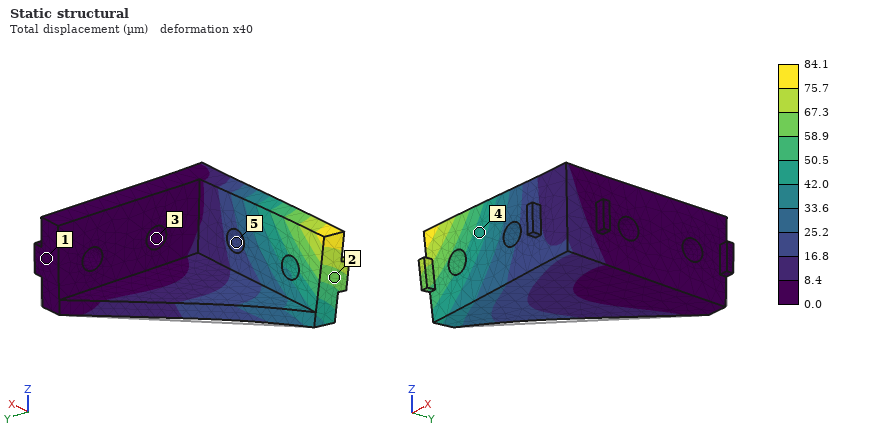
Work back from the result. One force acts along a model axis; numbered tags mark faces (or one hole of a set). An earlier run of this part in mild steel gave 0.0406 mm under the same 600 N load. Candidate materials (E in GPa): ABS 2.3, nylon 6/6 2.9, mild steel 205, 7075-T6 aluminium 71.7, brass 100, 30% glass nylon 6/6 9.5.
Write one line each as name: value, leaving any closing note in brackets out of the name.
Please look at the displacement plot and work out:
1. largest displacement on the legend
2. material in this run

largest displacement on the legend: 84.1 µm
material in this run: brass
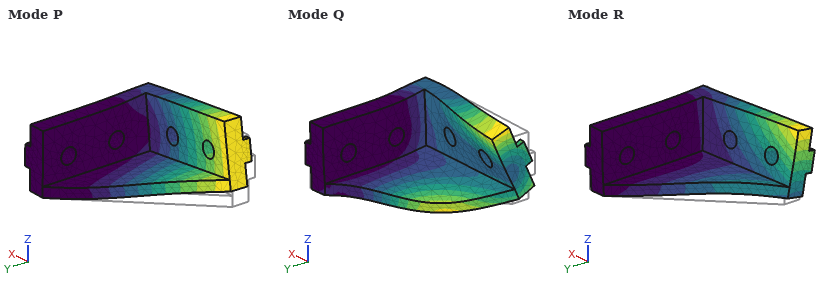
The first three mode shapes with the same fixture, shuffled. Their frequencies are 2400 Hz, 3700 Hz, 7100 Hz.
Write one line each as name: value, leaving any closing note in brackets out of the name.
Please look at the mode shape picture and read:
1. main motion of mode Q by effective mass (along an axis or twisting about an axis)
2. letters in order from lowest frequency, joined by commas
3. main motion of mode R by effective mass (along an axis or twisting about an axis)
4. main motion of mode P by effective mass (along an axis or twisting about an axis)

main motion of mode Q by effective mass: along X
letters in order from lowest frequency, joined by commas: P, R, Q
main motion of mode R by effective mass: along Y
main motion of mode P by effective mass: along Z
